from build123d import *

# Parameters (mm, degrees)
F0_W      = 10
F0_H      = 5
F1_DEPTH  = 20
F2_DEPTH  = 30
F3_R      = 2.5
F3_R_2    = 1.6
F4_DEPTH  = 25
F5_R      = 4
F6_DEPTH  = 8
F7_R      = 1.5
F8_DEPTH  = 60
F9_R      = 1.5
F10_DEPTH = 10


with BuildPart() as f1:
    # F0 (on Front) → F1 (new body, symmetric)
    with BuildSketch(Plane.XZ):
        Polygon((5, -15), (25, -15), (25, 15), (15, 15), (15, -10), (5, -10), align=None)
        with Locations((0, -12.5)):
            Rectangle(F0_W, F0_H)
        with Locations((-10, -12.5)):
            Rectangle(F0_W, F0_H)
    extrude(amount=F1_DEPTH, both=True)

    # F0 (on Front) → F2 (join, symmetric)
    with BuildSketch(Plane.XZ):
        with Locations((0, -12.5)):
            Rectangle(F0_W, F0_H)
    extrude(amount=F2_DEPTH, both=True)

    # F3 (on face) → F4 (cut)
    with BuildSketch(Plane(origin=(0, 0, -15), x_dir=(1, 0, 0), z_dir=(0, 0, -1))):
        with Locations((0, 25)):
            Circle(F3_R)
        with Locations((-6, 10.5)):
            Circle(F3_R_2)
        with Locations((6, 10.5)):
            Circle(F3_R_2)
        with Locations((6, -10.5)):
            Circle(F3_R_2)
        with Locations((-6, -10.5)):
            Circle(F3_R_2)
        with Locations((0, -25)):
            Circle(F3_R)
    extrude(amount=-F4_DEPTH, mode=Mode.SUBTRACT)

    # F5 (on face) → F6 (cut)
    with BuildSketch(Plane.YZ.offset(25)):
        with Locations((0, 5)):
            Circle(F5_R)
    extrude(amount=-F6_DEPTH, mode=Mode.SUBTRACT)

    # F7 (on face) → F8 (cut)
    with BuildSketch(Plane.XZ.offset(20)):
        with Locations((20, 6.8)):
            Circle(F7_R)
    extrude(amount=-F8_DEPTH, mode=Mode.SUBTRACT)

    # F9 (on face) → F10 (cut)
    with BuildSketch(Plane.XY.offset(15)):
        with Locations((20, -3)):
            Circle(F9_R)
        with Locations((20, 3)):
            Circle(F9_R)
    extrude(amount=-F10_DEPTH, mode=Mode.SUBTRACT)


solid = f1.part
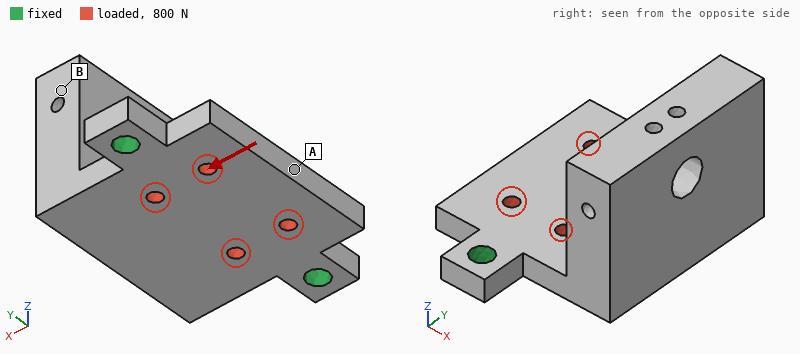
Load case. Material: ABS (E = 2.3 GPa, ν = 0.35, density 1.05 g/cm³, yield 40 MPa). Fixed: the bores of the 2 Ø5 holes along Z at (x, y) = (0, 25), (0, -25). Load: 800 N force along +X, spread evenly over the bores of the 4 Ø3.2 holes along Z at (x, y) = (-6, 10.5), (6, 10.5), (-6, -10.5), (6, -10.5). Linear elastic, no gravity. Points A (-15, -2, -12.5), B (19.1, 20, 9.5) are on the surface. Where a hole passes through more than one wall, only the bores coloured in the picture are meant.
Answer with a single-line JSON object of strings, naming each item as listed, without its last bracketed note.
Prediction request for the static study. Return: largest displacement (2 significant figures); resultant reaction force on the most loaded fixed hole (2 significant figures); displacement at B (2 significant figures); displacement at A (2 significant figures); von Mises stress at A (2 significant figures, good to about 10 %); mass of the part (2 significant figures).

{"largest displacement": "0.11 mm", "resultant reaction force on the most loaded fixed hole": "400 N", "displacement at B": "0.100 mm", "displacement at A": "0.11 mm", "von Mises stress at A": "4.9 MPa", "mass of the part": "19 g"}
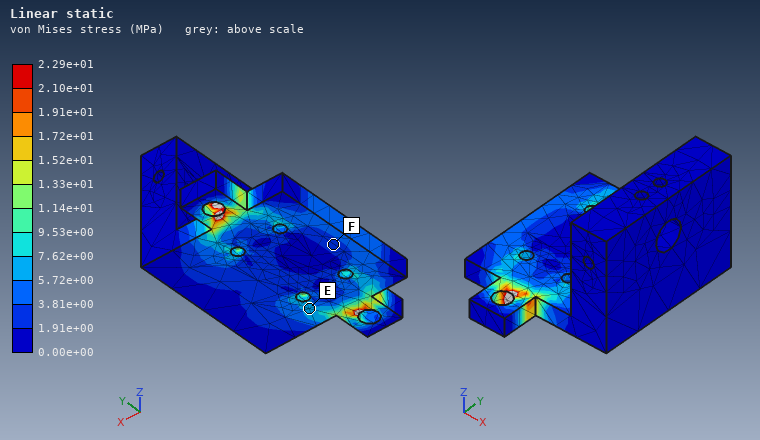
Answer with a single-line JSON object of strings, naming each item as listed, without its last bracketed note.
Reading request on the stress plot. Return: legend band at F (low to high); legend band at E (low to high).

{"legend band at F": "1.91e+00 to 3.81e+00 MPa", "legend band at E": "5.72e+00 to 7.62e+00 MPa"}
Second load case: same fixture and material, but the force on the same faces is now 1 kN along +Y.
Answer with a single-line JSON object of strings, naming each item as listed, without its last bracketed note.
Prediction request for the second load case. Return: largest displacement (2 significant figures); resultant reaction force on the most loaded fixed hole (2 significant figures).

{"largest displacement": "58 µm", "resultant reaction force on the most loaded fixed hole": "500 N"}
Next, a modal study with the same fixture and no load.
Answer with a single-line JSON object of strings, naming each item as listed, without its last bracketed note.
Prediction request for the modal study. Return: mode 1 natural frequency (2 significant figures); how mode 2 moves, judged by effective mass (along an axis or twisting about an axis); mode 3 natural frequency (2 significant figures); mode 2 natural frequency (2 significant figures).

{"mode 1 natural frequency": "400 Hz", "how mode 2 moves, judged by effective mass": "along Y", "mode 3 natural frequency": "1600 Hz", "mode 2 natural frequency": "1100 Hz"}
